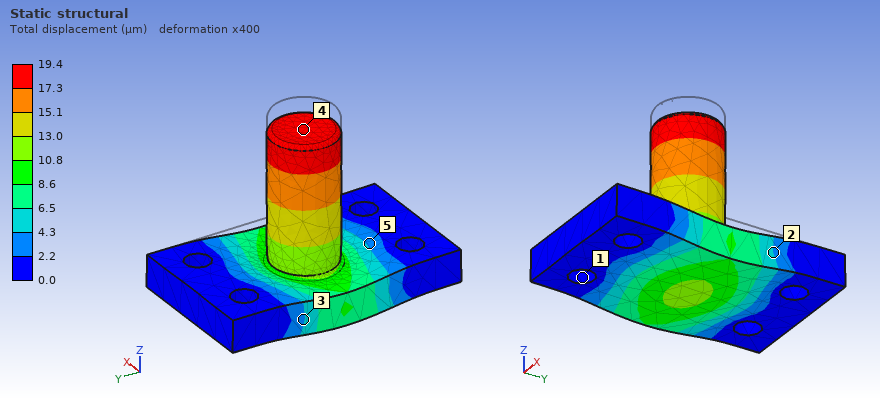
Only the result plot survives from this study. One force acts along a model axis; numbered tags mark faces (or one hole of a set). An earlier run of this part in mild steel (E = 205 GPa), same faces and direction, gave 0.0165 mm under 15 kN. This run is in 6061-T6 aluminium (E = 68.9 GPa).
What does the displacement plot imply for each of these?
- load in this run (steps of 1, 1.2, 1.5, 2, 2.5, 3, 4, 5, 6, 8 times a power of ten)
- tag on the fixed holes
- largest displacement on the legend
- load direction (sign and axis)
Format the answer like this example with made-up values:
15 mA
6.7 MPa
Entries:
6 kN
1
19.4 µm
-Z
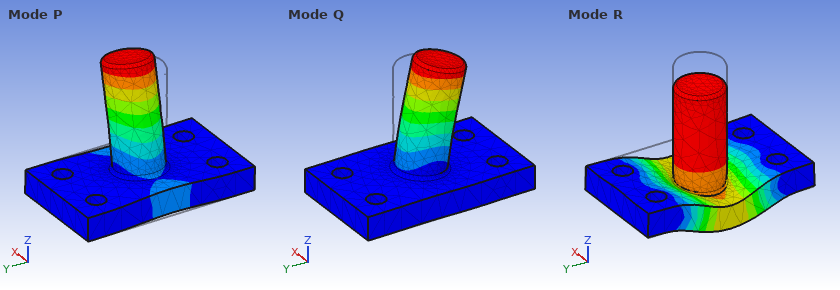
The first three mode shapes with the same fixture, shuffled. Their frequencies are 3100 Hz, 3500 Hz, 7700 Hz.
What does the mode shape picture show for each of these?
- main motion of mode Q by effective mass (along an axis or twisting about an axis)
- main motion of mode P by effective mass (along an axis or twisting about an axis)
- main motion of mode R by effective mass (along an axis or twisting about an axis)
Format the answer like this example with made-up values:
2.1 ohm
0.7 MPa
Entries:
along Y
along X
along Z
